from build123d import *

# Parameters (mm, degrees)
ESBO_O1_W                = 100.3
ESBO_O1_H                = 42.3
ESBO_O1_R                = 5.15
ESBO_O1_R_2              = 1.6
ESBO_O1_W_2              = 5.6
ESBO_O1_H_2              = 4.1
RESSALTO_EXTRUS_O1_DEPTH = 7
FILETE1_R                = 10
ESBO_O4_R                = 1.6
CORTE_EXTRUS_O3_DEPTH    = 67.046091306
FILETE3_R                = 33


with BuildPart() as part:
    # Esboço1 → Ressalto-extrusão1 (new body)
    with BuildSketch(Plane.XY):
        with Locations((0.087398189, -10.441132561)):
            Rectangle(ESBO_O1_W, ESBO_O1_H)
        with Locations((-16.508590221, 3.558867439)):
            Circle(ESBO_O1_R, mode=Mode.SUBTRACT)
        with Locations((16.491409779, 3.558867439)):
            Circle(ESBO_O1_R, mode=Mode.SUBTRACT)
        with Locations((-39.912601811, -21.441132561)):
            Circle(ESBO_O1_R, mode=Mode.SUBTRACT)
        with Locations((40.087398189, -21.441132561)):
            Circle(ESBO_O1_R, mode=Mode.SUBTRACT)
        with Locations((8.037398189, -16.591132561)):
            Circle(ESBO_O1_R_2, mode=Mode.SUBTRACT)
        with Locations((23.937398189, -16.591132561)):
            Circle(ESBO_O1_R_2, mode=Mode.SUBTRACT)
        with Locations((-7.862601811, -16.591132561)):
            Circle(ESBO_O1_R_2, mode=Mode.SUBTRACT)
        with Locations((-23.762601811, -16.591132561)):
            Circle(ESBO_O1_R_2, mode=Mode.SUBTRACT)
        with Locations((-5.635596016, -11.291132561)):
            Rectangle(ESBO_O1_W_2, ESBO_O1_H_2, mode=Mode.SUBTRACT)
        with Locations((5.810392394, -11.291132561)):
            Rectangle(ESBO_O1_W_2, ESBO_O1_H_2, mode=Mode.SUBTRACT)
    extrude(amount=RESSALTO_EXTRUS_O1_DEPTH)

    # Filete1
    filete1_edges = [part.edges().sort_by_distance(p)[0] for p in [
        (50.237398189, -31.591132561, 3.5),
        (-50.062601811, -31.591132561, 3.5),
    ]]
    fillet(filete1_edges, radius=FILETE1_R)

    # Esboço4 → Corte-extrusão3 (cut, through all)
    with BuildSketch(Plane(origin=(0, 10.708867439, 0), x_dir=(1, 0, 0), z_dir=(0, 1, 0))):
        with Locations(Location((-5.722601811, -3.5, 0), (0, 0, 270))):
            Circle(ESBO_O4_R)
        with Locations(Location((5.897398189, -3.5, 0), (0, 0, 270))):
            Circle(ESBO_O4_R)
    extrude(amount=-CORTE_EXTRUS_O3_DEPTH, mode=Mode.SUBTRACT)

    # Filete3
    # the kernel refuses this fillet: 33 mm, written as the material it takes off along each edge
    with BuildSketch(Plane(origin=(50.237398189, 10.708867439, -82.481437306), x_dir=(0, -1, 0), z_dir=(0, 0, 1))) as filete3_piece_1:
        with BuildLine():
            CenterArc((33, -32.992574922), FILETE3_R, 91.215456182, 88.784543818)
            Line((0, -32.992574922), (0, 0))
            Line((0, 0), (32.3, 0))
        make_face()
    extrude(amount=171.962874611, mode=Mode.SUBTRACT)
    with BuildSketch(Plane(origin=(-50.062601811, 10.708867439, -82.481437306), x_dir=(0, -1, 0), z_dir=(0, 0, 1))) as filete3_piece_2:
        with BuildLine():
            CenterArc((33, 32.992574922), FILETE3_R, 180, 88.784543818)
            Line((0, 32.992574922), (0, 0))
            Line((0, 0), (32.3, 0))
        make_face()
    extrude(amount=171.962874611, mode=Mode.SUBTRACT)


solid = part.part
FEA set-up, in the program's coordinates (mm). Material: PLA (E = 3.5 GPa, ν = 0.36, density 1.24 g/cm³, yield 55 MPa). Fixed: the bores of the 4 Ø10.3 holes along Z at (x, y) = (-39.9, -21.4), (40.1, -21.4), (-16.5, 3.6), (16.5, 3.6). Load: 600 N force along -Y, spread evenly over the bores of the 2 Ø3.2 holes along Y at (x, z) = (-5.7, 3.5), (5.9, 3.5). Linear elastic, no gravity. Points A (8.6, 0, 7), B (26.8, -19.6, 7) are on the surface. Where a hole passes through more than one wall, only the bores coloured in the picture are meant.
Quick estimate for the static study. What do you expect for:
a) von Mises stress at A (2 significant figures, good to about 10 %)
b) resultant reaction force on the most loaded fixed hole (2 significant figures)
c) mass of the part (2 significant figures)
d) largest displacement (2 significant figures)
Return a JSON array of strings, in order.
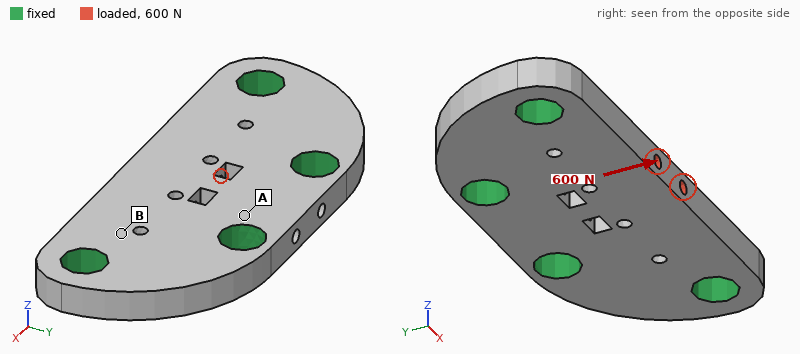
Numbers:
["2.2 MPa", "300 N", "28 g", "31 µm"]
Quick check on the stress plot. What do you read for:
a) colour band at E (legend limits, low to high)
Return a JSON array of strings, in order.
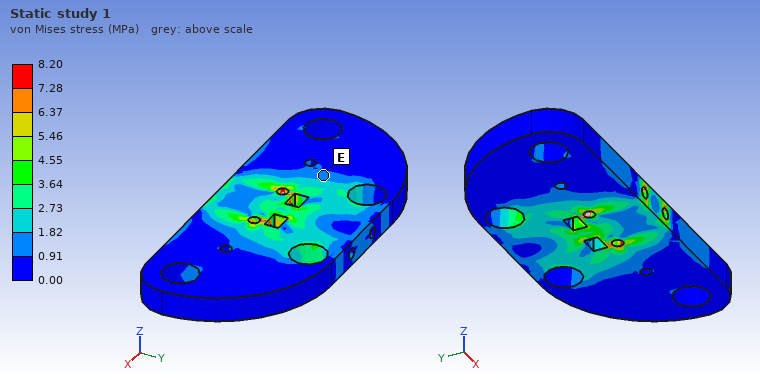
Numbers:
["0.91 to 1.82 MPa"]
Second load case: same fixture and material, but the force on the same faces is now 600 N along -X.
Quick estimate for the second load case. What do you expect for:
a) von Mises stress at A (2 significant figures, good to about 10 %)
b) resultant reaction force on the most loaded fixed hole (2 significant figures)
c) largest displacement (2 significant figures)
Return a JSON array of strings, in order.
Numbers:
["0.86 MPa", "210 N", "20 µm"]
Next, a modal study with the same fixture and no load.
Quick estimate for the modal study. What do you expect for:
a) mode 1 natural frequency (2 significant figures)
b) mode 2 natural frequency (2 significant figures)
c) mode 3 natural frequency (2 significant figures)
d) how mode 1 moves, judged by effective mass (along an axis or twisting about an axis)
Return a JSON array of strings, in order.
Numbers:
["3200 Hz", "6300 Hz", "8400 Hz", "along Z"]
